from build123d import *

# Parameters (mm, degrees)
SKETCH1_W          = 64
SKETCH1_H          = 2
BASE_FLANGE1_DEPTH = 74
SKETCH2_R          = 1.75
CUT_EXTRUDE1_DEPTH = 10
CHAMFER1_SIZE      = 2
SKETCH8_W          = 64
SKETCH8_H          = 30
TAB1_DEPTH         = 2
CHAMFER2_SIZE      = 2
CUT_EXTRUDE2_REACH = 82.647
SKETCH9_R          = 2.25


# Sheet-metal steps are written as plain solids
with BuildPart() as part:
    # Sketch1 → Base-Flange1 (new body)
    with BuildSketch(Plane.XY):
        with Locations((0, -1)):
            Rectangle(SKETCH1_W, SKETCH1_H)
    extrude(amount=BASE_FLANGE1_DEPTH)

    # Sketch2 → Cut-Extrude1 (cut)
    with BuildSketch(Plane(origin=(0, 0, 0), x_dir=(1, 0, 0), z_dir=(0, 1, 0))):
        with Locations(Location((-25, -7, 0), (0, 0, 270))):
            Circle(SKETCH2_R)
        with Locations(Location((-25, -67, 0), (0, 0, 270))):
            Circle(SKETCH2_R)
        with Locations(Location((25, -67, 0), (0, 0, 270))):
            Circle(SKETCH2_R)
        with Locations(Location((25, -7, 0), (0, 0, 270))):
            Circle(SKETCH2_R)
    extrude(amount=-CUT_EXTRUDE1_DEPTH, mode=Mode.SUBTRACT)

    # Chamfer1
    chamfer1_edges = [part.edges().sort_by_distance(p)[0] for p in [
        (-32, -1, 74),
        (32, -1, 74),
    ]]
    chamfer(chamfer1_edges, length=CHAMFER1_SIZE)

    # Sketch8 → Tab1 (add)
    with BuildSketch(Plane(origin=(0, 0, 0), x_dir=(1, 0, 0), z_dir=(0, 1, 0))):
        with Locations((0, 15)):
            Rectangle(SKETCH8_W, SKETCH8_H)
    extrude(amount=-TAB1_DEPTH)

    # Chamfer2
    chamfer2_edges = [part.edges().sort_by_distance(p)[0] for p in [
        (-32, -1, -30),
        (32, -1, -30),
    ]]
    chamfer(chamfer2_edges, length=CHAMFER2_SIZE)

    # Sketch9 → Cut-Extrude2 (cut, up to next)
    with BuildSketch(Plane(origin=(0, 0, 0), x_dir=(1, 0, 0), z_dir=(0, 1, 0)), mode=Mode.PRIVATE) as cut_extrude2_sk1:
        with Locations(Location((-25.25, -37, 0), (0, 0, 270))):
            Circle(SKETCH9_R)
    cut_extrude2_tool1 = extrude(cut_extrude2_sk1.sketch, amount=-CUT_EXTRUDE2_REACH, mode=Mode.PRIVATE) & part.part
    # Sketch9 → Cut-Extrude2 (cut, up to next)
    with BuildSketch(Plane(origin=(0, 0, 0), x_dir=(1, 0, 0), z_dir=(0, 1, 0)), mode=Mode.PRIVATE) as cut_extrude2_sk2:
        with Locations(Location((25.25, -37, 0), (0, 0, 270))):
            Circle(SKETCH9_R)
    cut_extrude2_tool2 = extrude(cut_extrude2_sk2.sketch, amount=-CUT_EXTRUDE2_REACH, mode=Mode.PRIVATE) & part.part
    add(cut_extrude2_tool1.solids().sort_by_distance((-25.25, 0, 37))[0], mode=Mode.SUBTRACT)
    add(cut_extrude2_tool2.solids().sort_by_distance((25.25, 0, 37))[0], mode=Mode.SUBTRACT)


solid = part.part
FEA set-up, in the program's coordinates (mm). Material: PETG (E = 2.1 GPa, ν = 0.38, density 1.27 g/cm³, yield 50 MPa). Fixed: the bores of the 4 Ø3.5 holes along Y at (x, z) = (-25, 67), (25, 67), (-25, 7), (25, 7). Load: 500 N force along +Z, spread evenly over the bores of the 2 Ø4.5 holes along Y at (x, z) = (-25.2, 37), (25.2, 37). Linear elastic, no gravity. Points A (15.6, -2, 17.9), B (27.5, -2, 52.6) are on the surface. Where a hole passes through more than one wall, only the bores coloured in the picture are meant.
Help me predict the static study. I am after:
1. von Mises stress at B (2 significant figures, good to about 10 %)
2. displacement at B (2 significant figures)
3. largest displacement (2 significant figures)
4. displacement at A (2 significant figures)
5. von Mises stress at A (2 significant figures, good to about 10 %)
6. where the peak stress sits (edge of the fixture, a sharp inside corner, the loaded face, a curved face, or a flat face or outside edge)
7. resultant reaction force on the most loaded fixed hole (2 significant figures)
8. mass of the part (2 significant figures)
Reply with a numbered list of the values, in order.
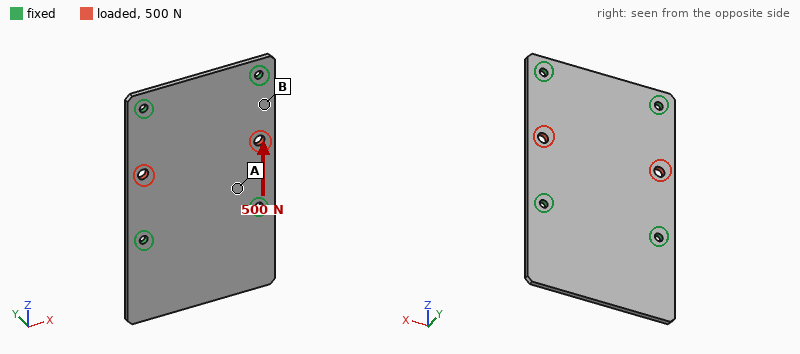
1. 4.0 MPa
2. 30 µm
3. 69 µm
4. 24 µm
5. 1.5 MPa
6. the loaded face
7. 130 N
8. 17 g
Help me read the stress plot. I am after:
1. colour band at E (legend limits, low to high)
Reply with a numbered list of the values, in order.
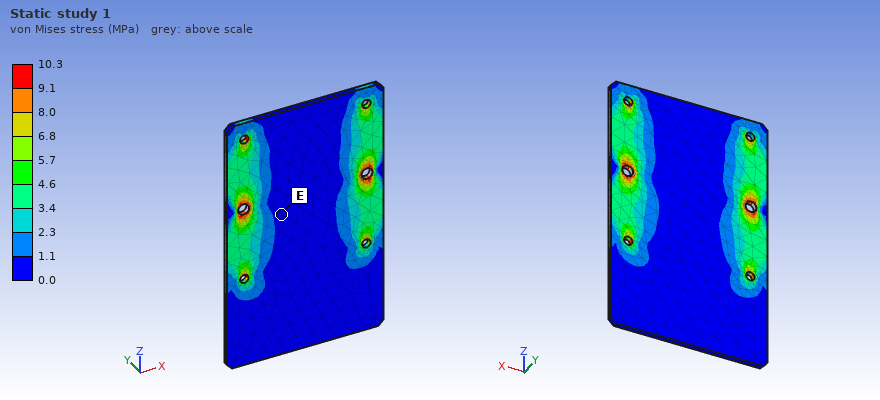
1. 0.0 to 1.1 MPa
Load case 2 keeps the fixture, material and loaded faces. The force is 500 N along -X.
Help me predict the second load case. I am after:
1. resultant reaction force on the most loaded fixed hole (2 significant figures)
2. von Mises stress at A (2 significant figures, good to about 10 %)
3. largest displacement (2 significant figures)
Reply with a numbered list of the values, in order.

1. 140 N
2. 4.5 MPa
3. 0.15 mm
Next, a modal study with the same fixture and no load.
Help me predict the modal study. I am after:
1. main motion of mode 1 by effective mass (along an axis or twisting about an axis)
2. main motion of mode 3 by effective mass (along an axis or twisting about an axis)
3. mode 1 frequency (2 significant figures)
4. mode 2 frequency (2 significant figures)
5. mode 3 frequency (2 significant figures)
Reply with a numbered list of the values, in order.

1. along Y
2. along Y
3. 270 Hz
4. 520 Hz
5. 610 Hz
